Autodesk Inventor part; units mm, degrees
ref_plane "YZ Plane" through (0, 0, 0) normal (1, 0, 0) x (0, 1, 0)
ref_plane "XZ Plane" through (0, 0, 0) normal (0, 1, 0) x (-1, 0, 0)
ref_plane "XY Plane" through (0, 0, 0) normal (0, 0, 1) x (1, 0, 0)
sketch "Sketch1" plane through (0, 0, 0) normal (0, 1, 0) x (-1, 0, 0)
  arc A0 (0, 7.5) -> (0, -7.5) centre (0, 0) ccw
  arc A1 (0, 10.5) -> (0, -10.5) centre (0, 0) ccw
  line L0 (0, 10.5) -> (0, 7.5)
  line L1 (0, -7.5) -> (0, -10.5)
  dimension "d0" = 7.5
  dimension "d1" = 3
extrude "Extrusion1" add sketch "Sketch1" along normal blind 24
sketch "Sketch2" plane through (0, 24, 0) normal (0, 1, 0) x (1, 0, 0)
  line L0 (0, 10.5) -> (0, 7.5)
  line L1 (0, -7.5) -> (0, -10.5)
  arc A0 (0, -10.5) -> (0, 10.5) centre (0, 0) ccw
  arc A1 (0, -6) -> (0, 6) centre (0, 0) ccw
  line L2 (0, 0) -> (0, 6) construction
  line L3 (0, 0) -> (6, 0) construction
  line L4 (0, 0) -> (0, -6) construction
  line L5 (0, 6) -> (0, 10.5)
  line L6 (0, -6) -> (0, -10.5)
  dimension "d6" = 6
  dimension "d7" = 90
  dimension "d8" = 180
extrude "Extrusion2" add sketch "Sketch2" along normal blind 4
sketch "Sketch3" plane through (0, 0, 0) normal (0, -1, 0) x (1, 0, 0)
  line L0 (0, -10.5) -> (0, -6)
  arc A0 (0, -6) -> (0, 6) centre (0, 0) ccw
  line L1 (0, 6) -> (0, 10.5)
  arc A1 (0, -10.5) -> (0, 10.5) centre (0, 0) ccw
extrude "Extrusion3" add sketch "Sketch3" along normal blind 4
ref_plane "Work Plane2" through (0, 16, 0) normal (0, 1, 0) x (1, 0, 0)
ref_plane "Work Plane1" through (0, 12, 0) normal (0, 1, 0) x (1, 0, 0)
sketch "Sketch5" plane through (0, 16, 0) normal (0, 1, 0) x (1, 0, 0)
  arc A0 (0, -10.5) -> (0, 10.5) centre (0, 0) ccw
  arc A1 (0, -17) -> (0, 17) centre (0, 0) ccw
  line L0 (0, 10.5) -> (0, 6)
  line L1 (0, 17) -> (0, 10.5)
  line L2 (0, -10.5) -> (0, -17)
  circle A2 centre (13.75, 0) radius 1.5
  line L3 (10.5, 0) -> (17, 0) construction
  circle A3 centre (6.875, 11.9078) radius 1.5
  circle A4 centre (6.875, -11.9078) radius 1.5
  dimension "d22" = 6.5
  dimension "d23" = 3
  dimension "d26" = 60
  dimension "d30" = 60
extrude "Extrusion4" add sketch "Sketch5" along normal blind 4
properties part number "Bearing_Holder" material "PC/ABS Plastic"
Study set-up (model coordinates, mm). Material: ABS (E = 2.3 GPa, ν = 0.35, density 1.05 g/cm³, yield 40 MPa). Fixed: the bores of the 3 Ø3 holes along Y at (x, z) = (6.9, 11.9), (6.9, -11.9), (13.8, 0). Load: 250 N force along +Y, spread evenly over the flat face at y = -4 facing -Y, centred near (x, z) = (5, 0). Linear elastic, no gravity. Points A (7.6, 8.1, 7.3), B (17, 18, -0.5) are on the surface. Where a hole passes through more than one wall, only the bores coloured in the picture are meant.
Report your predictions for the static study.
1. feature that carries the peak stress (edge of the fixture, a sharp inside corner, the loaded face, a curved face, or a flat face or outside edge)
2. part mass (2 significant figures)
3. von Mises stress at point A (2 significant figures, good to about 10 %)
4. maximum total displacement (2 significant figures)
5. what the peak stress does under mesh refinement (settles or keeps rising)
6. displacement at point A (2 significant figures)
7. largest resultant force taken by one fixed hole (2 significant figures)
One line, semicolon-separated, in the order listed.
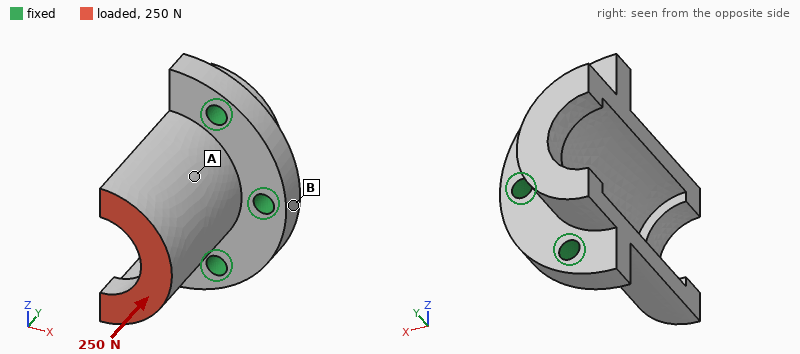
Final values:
edge of the fixture; 4.2 g; 2.8 MPa; 0.12 mm; keeps rising; 0.044 mm; 100 N
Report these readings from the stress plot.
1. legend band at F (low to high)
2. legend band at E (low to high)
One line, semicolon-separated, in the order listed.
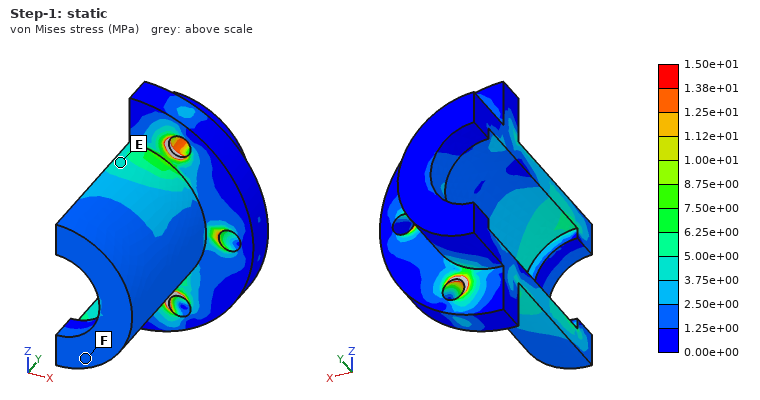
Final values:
1.25e+00 to 2.50e+00 MPa; 3.75e+00 to 5.00e+00 MPa
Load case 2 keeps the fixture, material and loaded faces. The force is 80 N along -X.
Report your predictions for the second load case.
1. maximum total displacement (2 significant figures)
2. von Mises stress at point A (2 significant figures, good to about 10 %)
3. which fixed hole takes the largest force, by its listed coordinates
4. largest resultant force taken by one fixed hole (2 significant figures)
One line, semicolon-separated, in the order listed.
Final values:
0.41 mm; 3.4 MPa; (13.8, 0); 150 N
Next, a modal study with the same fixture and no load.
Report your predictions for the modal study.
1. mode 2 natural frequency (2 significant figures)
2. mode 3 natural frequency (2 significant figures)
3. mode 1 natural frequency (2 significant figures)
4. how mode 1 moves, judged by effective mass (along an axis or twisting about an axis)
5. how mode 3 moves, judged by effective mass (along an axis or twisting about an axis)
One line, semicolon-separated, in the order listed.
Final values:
2900 Hz; 5100 Hz; 2700 Hz; along X; along Z
